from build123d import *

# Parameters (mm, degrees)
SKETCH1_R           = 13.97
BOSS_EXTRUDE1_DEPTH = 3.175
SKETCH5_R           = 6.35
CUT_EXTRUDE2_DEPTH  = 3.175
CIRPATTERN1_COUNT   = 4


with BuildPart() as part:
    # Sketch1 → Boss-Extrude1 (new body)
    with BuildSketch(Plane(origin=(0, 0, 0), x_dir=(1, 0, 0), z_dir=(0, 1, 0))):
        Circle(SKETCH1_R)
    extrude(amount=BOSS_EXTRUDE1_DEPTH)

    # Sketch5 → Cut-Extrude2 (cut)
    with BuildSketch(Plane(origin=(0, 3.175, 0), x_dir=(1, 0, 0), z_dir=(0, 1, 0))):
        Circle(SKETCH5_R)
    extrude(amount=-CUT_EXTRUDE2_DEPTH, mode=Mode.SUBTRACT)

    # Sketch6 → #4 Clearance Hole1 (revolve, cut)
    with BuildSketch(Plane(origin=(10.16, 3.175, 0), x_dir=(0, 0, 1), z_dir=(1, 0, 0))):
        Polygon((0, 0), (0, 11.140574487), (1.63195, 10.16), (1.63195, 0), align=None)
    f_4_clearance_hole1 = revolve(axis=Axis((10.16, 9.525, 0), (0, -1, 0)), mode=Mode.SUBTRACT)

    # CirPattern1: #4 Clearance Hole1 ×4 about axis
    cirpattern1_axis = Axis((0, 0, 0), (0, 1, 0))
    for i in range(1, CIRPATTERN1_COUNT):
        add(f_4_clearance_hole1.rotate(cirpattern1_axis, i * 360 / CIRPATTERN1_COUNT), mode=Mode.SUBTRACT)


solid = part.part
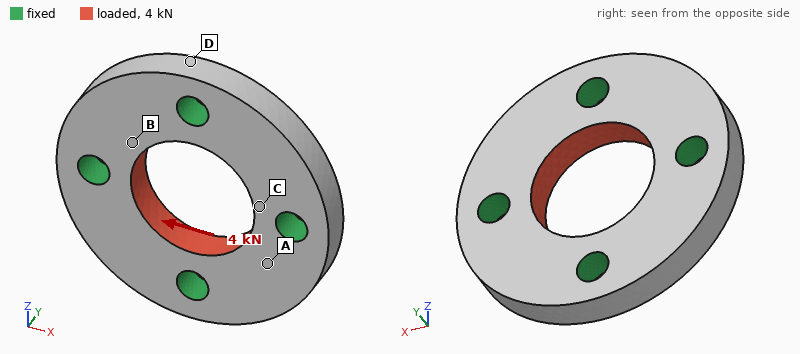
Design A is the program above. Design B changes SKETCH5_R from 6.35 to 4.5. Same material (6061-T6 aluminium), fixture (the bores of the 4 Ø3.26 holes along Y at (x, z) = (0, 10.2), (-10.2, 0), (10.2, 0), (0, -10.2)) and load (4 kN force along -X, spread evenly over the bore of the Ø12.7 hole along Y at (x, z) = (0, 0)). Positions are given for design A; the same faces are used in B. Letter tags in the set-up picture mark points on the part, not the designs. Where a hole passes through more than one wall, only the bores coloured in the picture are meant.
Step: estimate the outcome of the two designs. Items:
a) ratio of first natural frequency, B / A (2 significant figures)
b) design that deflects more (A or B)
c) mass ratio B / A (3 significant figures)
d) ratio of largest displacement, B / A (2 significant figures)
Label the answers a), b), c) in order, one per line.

a) 1.0
b) B
c) 1.14
d) 1.3
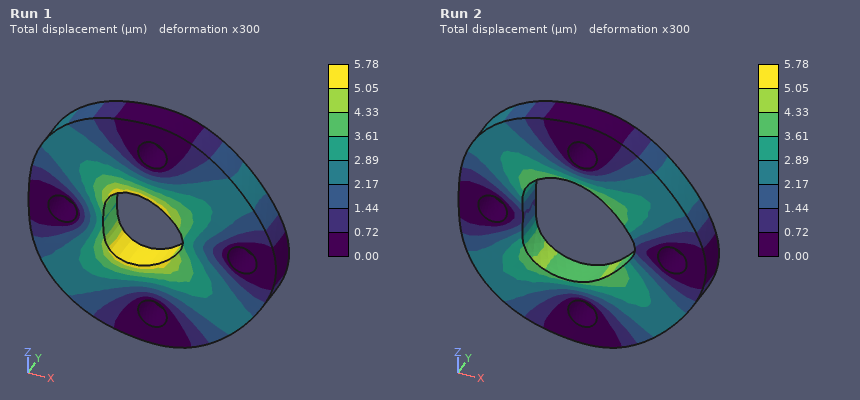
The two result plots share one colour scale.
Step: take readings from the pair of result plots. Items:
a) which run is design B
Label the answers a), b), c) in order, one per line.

a) Run 1
